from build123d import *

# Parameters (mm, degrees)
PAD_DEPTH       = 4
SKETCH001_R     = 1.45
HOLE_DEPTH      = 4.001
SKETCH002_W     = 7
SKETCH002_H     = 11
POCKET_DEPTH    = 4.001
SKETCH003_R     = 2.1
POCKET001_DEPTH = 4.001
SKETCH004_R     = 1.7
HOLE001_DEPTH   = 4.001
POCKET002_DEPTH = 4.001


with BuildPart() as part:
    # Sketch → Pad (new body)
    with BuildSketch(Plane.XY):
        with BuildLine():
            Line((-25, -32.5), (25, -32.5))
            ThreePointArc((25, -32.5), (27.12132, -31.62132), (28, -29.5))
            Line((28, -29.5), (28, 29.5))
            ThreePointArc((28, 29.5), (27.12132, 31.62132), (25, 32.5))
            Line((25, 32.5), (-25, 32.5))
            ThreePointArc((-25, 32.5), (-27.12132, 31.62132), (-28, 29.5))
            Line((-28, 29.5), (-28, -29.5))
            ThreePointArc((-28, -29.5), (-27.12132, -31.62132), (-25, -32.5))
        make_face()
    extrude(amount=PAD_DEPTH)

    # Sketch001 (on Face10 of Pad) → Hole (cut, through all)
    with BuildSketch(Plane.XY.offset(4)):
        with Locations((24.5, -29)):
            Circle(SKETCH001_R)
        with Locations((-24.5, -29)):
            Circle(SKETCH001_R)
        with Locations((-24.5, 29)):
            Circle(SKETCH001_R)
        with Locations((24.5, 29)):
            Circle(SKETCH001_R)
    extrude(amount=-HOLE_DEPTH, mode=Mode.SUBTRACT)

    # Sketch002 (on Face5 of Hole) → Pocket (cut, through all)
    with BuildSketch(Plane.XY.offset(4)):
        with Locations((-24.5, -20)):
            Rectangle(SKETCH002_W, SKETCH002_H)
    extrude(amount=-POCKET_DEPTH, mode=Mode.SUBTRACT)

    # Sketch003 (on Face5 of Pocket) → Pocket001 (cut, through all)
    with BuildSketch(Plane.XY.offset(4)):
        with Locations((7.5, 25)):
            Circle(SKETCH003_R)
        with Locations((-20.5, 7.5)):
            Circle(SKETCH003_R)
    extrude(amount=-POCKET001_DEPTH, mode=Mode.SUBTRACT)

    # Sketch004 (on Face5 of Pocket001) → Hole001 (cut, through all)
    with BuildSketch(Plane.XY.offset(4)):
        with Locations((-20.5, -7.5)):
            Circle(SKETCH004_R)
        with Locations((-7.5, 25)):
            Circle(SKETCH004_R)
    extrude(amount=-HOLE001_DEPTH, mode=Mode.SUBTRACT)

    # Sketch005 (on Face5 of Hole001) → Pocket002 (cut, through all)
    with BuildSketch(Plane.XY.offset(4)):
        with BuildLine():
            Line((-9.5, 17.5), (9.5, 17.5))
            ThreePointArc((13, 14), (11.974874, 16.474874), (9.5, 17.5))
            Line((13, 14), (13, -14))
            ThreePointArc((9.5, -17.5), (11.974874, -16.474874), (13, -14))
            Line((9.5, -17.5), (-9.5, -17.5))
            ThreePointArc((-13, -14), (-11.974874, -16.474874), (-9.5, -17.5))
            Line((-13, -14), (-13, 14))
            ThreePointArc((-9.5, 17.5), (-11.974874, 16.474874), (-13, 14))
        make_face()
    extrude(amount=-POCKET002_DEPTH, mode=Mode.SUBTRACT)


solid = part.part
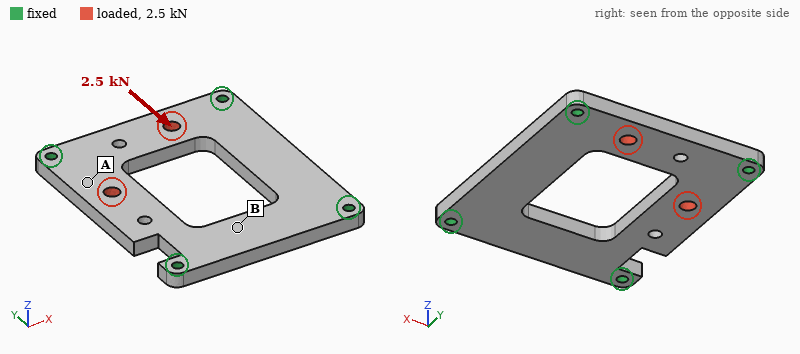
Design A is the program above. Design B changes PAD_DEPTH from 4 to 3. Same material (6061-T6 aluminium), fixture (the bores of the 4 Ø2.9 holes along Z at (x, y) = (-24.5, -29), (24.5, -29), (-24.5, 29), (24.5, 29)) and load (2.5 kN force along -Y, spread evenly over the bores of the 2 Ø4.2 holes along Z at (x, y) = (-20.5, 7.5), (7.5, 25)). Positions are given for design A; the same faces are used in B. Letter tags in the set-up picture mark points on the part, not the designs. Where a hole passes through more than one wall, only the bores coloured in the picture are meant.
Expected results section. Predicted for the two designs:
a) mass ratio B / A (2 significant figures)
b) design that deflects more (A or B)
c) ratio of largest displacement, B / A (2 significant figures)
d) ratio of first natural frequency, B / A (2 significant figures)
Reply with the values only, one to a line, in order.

0.75
B
1.3
0.78
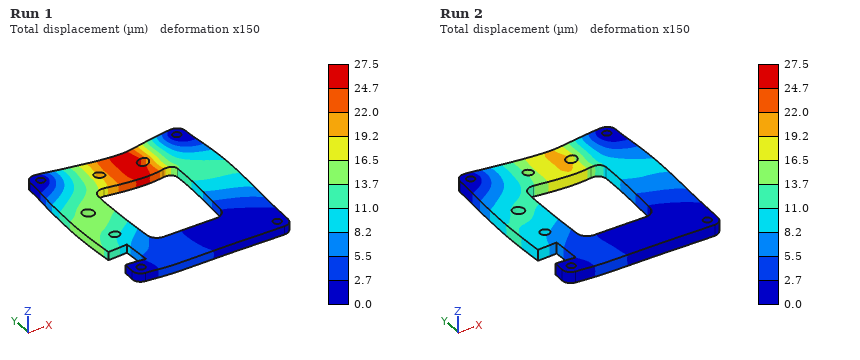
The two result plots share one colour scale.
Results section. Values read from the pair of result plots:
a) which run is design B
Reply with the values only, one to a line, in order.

Run 1
